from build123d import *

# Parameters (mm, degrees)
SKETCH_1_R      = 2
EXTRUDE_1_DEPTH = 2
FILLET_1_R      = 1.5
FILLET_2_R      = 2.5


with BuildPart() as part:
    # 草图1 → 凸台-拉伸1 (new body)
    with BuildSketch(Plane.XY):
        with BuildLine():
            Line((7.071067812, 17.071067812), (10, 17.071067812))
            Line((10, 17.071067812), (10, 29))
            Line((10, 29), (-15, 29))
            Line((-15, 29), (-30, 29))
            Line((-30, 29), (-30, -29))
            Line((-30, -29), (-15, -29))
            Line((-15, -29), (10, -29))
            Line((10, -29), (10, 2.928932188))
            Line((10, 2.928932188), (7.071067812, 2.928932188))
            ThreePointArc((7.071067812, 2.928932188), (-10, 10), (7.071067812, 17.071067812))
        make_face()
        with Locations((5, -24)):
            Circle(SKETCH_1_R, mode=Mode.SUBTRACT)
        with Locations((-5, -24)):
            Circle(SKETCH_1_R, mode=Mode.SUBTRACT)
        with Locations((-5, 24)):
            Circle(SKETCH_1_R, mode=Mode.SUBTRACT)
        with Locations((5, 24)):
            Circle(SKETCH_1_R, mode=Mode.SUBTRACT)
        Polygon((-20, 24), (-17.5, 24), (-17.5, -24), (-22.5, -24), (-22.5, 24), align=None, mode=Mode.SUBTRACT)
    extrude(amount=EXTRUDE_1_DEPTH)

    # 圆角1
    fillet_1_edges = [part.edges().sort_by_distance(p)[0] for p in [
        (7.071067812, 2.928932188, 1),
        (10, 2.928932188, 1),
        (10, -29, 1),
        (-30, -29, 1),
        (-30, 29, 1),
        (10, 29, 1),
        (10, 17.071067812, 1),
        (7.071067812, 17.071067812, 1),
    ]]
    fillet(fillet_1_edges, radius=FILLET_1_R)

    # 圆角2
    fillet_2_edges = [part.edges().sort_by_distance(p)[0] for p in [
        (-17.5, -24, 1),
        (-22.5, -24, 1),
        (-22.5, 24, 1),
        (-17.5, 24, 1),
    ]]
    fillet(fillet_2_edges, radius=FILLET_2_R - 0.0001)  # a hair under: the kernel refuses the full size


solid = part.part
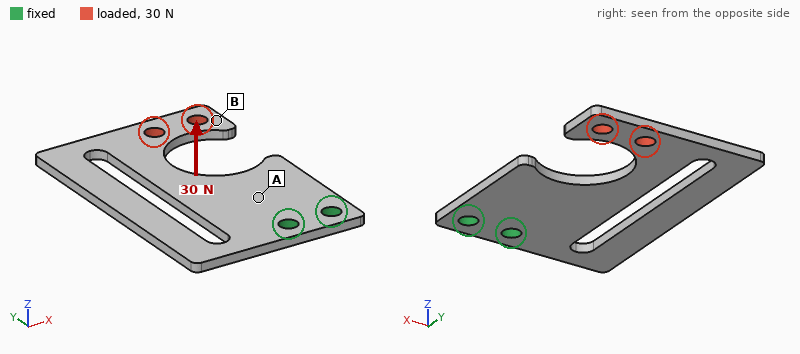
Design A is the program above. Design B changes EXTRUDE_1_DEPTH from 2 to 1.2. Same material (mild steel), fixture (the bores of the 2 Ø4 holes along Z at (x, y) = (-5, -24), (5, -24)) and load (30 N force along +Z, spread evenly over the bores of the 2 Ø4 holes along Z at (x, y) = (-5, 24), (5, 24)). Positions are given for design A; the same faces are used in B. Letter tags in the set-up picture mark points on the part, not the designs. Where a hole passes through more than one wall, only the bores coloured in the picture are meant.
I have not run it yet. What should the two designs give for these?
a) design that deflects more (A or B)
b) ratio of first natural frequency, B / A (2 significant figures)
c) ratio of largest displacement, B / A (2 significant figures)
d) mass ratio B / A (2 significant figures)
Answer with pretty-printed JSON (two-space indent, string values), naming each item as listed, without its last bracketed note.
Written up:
{
  "design that deflects more": "B",
  "ratio of first natural frequency, B / A": "0.61",
  "ratio of largest displacement, B / A": "4.5",
  "mass ratio B / A": "0.60"
}
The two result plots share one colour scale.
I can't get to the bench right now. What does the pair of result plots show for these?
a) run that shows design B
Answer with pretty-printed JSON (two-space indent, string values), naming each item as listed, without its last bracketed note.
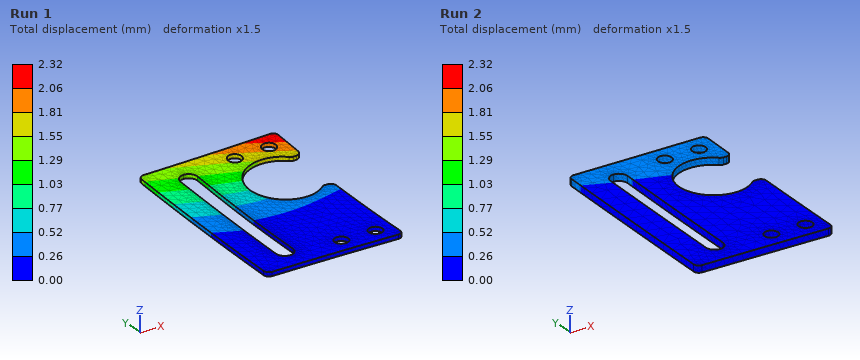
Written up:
{
  "run that shows design B": "Run 1"
}
